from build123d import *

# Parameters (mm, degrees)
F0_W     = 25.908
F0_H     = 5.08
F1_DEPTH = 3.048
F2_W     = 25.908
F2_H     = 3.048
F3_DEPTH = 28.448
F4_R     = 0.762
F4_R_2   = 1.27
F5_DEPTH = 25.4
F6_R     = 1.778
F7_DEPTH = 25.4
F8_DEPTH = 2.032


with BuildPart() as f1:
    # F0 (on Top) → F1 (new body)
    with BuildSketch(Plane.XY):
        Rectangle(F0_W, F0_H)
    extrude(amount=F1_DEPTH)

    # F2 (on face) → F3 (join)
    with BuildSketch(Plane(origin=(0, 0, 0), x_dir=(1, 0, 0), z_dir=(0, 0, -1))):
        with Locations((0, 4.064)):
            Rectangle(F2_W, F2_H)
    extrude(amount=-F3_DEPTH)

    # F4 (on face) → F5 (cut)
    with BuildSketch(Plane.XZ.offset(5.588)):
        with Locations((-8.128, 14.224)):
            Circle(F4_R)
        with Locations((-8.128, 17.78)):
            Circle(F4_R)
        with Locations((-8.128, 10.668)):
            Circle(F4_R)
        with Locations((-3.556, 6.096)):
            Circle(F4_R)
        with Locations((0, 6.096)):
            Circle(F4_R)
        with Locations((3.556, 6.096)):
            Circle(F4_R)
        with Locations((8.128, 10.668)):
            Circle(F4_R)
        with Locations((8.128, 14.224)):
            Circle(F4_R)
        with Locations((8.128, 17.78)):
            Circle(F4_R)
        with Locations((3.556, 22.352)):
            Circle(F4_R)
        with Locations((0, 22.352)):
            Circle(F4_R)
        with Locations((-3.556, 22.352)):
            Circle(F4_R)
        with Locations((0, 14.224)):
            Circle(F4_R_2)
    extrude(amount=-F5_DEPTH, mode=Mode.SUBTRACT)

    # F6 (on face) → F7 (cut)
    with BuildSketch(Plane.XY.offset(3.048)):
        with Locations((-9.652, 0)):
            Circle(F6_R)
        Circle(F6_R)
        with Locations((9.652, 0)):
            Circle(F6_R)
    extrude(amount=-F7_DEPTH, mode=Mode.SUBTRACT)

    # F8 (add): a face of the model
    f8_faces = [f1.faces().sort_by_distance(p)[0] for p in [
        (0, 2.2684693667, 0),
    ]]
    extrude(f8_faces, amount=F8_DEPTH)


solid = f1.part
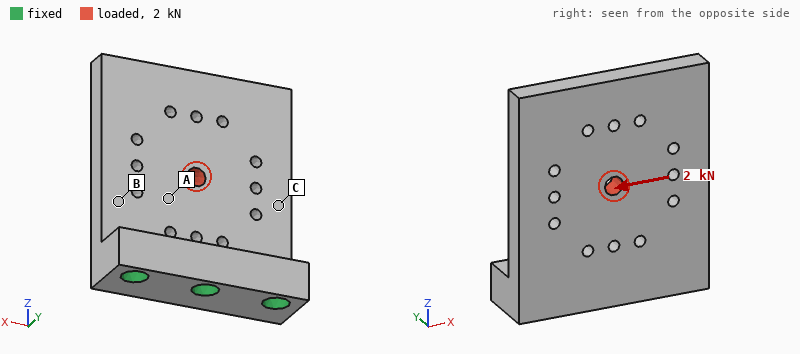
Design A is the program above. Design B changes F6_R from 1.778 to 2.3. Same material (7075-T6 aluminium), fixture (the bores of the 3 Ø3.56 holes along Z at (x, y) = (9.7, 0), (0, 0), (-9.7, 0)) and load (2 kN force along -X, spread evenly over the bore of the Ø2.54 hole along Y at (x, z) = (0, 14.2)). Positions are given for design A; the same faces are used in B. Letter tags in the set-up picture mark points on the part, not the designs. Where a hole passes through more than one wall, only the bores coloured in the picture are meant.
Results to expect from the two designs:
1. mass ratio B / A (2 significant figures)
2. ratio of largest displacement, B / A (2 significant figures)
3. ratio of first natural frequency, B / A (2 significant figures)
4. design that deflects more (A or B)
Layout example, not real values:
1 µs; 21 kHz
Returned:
0.96; 0.87; 1.0; A
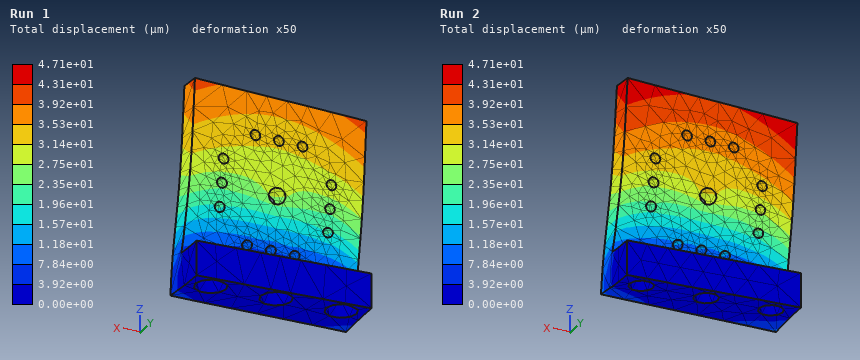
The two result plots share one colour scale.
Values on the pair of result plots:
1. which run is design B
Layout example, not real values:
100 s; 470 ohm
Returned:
Run 1
